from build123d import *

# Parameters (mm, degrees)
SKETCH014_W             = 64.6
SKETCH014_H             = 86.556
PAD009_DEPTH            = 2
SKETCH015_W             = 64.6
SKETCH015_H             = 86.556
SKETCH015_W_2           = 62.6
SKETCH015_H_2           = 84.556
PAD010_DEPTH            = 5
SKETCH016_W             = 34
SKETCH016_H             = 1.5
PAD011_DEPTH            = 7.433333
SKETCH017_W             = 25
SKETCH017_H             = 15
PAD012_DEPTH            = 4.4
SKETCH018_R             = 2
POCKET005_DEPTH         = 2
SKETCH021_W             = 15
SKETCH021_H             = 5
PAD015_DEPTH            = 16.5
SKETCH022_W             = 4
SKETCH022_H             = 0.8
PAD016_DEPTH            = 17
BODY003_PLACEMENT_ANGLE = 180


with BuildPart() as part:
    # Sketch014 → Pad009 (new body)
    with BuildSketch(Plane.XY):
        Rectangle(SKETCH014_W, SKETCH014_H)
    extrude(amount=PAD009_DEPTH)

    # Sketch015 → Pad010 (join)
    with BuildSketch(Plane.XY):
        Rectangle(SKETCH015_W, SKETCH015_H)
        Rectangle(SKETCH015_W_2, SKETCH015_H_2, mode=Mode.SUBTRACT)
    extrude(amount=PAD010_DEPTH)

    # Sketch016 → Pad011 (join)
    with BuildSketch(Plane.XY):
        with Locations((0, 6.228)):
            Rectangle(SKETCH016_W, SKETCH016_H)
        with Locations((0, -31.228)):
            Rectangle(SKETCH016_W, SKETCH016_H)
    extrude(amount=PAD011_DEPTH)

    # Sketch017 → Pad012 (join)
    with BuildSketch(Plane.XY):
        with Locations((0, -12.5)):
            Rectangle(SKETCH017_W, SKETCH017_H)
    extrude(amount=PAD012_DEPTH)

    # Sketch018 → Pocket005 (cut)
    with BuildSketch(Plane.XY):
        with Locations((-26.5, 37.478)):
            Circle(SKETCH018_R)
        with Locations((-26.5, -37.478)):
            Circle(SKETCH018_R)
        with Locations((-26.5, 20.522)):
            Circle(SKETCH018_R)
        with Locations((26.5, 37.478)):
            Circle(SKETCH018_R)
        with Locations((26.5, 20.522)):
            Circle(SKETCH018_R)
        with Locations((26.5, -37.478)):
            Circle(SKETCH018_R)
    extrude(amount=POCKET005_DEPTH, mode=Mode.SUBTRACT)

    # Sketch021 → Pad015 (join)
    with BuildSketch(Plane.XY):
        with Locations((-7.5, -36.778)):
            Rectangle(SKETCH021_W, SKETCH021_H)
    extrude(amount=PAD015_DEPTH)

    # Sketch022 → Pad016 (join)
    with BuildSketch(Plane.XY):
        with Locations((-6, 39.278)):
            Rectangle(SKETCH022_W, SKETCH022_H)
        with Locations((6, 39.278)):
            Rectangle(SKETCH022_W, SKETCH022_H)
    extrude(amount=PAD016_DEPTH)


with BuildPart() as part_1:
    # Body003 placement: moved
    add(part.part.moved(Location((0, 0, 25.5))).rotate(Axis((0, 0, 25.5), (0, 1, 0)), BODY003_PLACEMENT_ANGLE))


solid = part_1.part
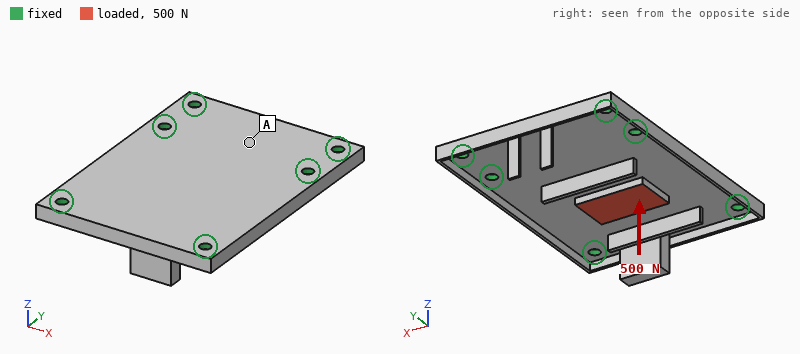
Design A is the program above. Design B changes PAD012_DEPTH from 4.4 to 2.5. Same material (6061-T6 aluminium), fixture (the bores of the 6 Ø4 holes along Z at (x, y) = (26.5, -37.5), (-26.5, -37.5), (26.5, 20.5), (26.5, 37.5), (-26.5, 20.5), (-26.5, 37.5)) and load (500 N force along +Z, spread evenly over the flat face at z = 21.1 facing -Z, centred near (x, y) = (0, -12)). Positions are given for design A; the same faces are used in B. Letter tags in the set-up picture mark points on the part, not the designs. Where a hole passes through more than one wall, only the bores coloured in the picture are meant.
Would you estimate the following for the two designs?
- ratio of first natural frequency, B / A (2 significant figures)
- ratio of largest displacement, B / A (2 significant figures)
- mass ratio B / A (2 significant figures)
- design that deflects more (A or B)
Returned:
1.0
1.3
0.95
B
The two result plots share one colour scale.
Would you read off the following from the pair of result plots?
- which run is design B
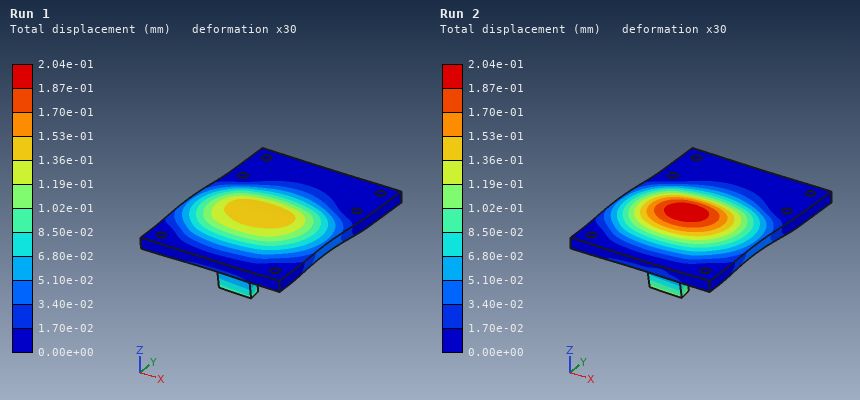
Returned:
Run 2
